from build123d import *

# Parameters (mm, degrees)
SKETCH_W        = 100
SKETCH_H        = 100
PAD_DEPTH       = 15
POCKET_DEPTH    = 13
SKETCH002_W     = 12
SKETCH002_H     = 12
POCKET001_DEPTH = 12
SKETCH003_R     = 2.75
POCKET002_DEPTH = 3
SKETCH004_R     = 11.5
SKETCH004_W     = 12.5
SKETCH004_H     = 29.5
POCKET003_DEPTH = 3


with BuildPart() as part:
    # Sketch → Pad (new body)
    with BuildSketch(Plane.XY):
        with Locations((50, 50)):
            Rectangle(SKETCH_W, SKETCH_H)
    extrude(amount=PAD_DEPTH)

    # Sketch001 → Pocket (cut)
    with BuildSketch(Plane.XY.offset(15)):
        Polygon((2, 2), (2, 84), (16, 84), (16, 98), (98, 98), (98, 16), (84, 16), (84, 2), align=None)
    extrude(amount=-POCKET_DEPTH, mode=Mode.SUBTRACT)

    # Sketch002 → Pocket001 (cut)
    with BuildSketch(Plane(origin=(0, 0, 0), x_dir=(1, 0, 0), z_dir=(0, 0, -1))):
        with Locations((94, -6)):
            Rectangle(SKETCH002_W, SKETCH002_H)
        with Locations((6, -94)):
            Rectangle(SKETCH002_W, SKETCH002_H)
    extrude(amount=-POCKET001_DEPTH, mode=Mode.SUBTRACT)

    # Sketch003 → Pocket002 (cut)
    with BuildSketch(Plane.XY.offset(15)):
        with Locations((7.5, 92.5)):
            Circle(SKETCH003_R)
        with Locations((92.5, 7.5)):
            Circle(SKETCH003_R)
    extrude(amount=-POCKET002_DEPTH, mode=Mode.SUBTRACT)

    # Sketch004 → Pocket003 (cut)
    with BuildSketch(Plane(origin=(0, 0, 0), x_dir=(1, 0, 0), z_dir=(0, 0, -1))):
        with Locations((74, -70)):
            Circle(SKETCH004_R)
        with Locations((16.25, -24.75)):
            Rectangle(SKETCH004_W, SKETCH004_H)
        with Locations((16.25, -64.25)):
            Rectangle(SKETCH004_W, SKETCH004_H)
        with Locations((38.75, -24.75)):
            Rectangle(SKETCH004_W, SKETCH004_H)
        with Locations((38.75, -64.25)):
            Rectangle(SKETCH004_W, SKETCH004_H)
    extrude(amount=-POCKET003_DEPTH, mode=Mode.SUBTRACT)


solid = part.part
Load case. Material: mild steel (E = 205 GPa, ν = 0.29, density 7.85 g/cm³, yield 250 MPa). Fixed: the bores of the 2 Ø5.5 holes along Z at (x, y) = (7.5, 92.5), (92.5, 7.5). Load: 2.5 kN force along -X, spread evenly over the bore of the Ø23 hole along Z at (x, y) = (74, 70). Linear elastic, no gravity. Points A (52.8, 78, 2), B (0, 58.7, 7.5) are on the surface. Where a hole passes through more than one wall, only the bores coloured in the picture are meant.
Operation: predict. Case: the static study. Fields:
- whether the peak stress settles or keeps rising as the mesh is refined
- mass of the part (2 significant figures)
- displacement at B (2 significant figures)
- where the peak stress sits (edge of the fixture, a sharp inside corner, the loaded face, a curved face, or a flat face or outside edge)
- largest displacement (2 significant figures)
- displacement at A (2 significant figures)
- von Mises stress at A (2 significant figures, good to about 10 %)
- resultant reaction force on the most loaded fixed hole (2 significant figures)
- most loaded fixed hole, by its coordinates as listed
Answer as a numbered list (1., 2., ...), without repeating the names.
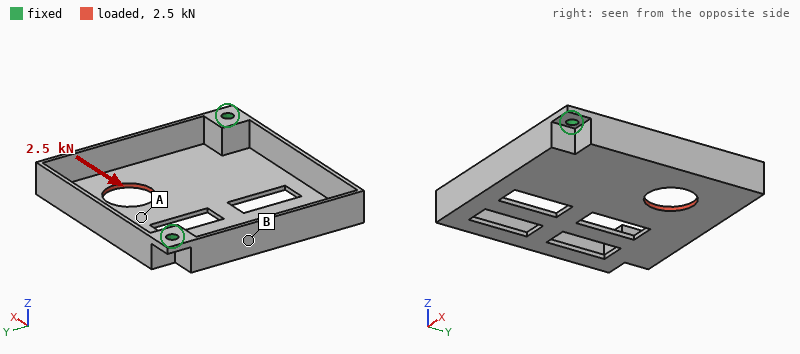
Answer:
1. keeps rising
2. 220 g
3. 0.050 mm
4. edge of the fixture
5. 0.16 mm
6. 0.057 mm
7. 31 MPa
8. 1.6 kN
9. (7.5, 92.5)
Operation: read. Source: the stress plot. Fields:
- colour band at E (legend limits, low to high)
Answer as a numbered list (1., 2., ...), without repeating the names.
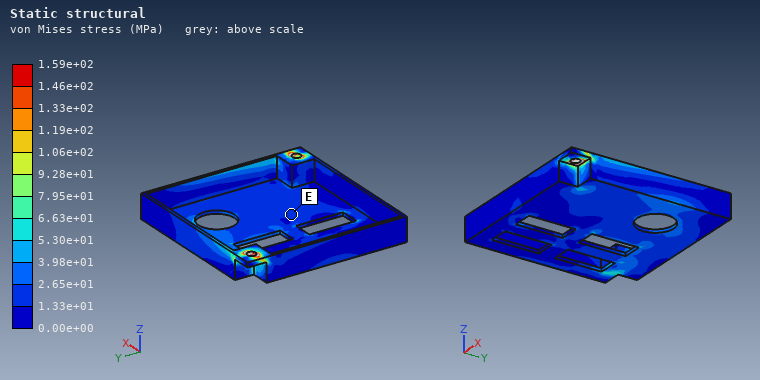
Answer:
1. 1.33e+01 to 2.65e+01 MPa
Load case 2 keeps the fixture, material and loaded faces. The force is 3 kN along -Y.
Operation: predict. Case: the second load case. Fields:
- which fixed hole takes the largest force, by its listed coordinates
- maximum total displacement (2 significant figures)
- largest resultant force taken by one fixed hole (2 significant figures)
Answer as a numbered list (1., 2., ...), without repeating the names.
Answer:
1. (92.5, 7.5)
2. 0.20 mm
3. 2.0 kN
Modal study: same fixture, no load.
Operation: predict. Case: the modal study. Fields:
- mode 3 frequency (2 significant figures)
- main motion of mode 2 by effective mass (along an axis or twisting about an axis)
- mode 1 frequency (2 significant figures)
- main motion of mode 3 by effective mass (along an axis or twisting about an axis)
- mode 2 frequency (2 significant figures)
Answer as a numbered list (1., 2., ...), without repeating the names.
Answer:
1. 1800 Hz
2. along Z
3. 930 Hz
4. along Z
5. 1200 Hz
